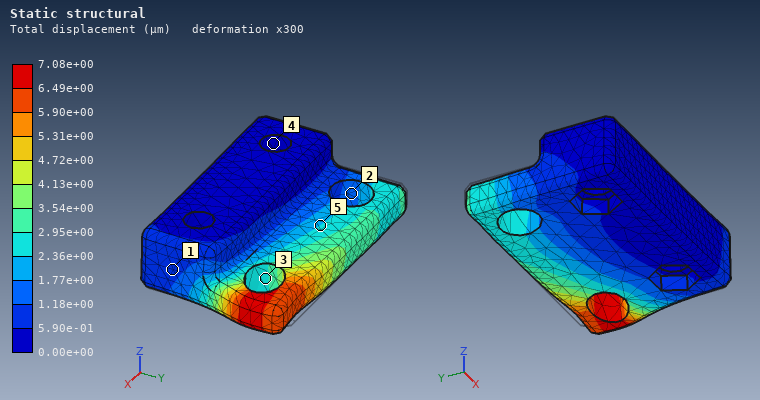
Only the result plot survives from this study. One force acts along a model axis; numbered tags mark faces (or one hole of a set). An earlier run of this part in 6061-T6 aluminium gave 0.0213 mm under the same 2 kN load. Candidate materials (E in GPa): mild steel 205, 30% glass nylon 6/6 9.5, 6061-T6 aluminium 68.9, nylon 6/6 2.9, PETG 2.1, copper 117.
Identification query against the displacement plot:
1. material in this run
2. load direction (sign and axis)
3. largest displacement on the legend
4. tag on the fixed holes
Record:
mild steel
+X
7.08e+00 µm
4
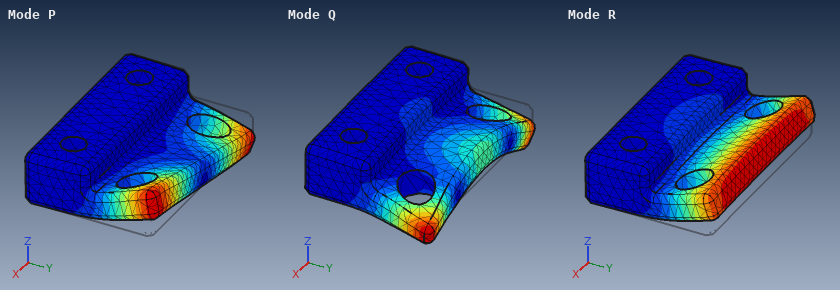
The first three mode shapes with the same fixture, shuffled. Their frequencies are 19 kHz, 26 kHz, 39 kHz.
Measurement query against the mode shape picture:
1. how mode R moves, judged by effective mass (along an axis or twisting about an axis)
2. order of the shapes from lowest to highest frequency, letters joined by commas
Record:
along Z
R, P, Q
